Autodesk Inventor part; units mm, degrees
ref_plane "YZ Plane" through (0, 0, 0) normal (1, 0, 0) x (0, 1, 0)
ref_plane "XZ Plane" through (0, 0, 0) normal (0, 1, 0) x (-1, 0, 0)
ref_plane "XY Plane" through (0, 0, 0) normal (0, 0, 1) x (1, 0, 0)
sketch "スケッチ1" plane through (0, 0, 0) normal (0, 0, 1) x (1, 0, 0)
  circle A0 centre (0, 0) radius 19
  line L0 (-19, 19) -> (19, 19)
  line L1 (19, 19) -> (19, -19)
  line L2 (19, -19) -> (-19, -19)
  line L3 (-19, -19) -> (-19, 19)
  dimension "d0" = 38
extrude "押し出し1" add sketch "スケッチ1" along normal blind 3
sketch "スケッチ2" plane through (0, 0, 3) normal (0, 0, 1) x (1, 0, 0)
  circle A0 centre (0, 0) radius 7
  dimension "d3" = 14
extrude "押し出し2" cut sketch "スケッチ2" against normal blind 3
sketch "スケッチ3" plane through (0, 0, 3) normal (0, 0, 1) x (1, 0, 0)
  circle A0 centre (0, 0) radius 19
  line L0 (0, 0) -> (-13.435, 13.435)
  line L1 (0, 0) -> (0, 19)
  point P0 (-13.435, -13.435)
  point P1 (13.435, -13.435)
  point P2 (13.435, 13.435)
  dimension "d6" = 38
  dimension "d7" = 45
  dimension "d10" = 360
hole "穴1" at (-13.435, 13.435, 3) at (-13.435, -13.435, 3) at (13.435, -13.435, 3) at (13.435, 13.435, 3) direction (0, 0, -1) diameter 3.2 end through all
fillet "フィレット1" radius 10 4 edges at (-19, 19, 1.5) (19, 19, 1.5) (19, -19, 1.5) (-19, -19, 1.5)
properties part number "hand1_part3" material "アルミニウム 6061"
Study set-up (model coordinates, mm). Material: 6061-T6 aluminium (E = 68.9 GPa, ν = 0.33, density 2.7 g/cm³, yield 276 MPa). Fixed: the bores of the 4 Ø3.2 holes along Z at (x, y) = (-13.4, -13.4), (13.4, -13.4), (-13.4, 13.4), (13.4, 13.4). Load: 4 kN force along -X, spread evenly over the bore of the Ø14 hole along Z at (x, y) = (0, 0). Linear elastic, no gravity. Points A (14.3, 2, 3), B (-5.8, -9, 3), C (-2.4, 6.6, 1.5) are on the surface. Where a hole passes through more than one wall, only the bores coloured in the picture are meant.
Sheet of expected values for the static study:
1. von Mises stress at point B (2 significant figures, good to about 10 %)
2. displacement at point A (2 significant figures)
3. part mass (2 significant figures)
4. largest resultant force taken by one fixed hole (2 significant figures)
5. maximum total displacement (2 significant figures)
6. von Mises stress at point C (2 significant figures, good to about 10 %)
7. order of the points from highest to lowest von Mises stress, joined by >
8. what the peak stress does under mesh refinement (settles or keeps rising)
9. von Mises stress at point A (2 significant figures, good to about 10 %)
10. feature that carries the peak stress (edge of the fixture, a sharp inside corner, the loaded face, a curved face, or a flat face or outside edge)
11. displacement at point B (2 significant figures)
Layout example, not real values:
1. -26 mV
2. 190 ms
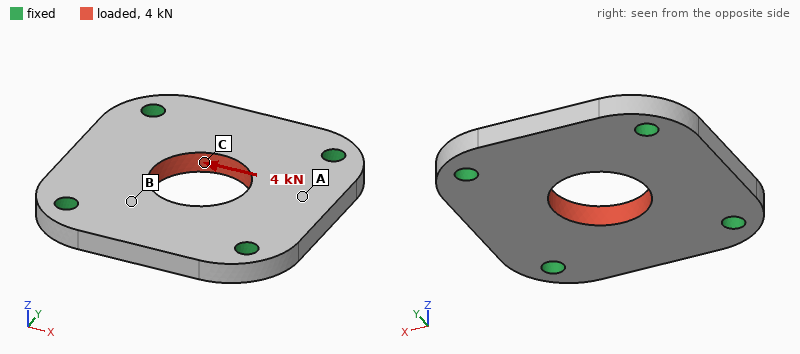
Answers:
1. 34 MPa
2. 8.5 µm
3. 9.5 g
4. 1.1 kN
5. 11 µm
6. 55 MPa
7. C > B > A
8. keeps rising
9. 15 MPa
10. edge of the fixture
11. 5.0 µm
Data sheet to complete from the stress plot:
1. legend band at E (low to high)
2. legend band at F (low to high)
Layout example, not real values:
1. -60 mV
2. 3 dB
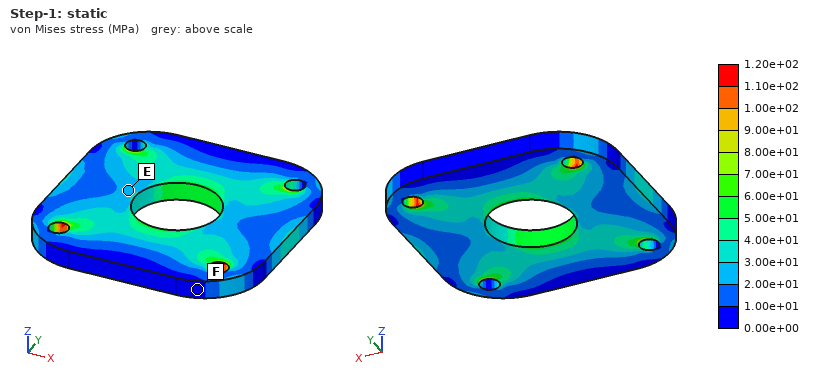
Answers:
1. 2.00e+01 to 3.00e+01 MPa
2. 0.00e+00 to 1.00e+01 MPa
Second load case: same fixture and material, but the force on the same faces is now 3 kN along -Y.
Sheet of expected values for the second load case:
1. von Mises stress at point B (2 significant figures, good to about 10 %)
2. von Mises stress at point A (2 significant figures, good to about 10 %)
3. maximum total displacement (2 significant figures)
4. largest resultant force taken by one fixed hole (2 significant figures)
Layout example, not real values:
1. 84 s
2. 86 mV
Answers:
1. 24 MPa
2. 11 MPa
3. 8.1 µm
4. 790 N
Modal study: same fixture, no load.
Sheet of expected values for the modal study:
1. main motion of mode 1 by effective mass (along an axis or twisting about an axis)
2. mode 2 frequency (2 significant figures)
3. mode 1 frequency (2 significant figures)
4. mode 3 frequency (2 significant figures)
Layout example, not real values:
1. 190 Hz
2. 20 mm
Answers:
1. along Z
2. 22 kHz
3. 18 kHz
4. 22 kHz
